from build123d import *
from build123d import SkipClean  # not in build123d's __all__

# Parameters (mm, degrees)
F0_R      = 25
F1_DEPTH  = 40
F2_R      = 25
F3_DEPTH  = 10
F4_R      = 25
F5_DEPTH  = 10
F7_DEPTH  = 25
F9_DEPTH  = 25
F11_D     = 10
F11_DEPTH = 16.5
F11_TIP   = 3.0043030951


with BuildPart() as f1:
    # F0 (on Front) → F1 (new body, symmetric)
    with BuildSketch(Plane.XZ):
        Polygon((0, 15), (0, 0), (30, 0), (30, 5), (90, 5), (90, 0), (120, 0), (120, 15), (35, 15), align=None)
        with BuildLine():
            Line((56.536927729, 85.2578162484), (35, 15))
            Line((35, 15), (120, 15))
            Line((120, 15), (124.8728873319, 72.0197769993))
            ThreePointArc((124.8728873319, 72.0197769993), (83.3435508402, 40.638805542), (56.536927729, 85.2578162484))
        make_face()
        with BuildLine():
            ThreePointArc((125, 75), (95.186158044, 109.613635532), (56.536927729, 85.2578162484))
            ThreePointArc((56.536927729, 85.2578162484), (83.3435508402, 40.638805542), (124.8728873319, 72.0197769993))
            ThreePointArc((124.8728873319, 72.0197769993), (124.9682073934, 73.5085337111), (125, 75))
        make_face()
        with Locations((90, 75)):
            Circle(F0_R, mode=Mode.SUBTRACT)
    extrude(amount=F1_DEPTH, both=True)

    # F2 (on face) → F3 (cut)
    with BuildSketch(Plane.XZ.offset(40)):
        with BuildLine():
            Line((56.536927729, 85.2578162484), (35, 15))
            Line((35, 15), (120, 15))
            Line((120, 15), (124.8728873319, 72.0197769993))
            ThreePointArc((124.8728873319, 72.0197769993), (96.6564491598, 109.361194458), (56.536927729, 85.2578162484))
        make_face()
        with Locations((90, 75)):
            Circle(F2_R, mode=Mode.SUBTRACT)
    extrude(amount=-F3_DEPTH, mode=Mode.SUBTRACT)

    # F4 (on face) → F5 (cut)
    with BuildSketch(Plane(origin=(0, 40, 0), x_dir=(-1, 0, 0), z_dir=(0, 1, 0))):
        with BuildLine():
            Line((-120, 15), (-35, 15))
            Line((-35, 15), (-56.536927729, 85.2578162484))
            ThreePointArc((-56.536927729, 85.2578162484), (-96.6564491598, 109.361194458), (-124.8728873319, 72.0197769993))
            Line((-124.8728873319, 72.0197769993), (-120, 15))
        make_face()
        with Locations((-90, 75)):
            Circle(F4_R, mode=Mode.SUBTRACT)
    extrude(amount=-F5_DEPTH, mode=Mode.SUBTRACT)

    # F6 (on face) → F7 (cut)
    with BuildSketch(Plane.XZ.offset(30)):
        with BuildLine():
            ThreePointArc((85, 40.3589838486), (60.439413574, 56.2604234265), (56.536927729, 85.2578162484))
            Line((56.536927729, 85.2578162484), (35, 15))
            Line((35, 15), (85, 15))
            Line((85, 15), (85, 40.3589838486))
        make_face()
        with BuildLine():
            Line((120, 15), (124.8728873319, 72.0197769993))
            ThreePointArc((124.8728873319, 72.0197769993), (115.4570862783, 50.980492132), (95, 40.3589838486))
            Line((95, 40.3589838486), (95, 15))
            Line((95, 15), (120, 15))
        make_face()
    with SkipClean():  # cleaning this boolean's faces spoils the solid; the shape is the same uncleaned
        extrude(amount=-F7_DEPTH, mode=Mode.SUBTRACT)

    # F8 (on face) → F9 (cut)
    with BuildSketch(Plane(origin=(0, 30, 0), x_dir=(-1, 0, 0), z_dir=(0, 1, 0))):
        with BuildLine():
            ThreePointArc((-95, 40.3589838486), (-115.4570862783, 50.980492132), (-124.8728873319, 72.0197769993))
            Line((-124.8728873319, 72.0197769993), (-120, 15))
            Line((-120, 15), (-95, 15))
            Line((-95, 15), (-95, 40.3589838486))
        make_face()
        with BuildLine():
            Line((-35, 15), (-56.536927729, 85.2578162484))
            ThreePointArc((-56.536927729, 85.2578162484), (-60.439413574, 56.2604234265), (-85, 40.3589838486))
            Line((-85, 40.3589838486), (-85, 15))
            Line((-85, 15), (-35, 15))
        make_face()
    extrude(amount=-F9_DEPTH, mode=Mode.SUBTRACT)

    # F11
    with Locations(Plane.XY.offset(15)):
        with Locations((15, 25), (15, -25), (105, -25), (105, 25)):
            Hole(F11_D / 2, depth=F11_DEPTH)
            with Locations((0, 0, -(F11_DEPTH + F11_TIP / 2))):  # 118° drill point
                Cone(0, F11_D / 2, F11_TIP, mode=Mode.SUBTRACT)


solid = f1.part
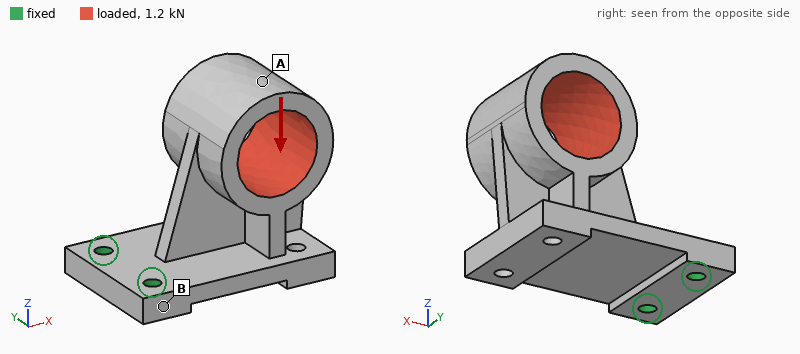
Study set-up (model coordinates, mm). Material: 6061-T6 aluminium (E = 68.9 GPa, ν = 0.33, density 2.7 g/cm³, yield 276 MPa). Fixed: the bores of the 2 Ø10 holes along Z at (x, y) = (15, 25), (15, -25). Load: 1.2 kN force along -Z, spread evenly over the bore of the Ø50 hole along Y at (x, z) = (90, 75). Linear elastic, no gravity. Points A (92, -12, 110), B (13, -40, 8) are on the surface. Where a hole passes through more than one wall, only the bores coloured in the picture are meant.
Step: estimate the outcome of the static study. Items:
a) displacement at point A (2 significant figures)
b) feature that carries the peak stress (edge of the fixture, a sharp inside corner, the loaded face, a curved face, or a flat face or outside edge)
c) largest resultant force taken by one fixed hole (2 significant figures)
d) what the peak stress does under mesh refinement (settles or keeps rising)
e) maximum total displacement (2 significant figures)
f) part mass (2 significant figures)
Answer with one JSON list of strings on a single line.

["0.41 mm", "edge of the fixture", "600 N", "keeps rising", "0.43 mm", "730 g"]
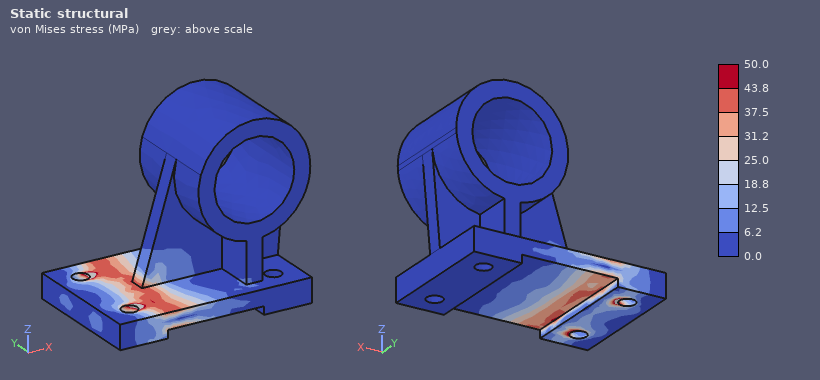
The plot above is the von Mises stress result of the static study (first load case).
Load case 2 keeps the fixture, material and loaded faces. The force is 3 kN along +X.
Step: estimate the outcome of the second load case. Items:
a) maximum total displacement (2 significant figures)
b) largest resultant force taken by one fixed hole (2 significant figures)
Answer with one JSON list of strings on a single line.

["1.3 mm", "1.7 kN"]
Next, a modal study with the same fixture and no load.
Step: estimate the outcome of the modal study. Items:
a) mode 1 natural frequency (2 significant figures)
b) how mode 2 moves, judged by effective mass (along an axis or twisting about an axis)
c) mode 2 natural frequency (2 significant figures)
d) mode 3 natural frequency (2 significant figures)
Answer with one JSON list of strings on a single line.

["370 Hz", "along Y", "590 Hz", "2400 Hz"]
